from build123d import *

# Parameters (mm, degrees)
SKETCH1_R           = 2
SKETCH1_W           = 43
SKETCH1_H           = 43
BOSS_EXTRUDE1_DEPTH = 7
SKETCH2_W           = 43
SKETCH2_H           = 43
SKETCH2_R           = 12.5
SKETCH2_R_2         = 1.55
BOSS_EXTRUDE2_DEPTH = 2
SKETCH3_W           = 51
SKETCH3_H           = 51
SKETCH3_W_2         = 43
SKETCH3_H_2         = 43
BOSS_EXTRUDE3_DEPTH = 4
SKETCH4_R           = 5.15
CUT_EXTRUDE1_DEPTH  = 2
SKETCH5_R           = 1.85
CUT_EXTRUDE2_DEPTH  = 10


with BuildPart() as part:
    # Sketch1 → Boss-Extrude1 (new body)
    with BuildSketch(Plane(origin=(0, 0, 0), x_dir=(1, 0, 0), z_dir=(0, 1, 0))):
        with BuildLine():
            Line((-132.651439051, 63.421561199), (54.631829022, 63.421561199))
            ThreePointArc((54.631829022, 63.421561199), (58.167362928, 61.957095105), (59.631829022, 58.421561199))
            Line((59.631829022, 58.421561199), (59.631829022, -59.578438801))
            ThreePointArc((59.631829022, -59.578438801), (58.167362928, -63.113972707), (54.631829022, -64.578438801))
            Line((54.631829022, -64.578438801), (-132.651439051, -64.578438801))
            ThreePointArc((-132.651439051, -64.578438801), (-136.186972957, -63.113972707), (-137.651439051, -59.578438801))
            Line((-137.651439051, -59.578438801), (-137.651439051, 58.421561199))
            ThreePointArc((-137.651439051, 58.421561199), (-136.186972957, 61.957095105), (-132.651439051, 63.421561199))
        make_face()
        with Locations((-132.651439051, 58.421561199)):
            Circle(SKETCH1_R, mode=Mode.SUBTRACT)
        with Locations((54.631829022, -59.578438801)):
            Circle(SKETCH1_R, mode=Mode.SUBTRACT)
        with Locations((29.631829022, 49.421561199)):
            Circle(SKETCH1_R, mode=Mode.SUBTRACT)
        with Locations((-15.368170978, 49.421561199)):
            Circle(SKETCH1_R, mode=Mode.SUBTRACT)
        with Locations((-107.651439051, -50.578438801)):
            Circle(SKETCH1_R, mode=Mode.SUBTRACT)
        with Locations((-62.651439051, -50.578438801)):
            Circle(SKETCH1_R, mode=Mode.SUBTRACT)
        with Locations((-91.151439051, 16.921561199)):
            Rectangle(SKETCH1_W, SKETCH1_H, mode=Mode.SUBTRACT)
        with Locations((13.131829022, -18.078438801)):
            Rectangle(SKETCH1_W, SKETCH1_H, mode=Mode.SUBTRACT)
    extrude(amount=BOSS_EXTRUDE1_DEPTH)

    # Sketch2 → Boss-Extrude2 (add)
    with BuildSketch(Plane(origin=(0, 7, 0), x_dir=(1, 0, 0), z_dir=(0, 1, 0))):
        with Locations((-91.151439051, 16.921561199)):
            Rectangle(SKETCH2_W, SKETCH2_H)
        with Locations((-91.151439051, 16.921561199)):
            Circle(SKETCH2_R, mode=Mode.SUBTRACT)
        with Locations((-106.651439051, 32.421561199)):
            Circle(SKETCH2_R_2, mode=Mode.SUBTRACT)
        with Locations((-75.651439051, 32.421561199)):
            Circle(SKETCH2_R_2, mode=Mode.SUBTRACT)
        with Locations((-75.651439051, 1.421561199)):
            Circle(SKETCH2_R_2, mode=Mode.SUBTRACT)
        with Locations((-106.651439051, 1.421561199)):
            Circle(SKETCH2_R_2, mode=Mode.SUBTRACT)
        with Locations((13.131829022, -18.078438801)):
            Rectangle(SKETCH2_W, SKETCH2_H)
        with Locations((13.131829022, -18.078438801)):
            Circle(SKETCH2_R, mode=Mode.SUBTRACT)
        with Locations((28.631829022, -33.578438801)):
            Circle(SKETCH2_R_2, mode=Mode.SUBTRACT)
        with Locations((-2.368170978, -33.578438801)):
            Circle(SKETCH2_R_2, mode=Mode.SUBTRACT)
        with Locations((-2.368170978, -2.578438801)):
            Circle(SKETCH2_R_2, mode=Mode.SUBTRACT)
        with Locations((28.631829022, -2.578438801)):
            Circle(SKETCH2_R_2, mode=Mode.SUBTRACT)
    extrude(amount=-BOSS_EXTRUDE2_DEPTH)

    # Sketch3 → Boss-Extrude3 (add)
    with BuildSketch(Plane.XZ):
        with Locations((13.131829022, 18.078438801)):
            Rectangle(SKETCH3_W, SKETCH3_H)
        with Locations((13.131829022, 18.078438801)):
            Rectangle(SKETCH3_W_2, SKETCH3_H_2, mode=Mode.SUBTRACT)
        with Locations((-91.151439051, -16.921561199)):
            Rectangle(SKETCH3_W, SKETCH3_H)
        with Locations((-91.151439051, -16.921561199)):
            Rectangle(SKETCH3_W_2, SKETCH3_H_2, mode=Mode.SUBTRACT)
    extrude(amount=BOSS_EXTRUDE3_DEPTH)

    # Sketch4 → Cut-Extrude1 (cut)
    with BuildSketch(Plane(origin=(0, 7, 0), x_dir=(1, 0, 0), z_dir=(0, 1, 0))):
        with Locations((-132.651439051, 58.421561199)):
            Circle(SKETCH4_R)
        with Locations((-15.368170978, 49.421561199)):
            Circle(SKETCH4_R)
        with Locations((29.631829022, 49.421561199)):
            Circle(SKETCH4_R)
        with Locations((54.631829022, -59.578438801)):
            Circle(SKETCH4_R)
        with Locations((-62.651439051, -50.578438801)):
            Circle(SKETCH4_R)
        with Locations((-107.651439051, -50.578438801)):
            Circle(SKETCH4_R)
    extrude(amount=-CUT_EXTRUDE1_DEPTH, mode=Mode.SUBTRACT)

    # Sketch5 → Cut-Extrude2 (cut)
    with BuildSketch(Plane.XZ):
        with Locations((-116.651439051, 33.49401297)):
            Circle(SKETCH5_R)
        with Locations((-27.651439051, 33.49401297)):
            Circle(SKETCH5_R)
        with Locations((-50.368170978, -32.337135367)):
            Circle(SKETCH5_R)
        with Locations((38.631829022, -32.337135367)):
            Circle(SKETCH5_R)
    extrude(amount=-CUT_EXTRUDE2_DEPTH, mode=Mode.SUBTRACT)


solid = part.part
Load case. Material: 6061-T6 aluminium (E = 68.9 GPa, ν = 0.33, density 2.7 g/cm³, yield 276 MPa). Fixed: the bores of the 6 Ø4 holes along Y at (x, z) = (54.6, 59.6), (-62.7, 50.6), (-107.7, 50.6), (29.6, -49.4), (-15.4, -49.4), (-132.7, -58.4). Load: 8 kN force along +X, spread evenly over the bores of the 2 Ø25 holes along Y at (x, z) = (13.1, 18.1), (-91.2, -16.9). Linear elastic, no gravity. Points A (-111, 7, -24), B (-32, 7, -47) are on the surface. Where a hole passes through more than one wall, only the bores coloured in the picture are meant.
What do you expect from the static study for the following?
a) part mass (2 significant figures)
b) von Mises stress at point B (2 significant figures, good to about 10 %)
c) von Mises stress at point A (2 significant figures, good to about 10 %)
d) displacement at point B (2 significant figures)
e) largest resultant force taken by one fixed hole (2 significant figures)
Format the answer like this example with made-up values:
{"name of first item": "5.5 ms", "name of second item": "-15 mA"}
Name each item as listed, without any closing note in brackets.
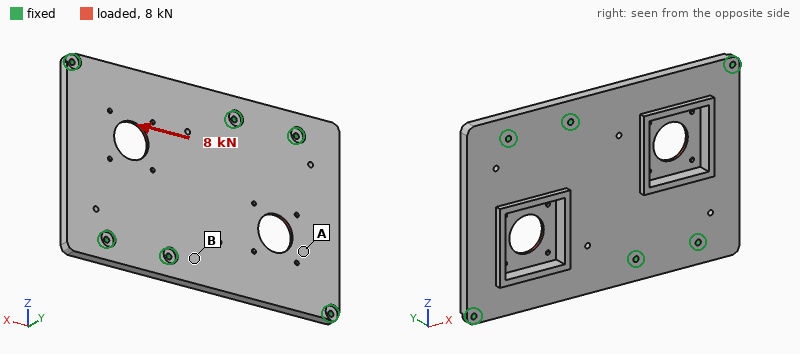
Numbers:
{"part mass": "430 g", "von Mises stress at point B": "7.3 MPa", "von Mises stress at point A": "18 MPa", "displacement at point B": "3.3 µm", "largest resultant force taken by one fixed hole": "1.9 kN"}
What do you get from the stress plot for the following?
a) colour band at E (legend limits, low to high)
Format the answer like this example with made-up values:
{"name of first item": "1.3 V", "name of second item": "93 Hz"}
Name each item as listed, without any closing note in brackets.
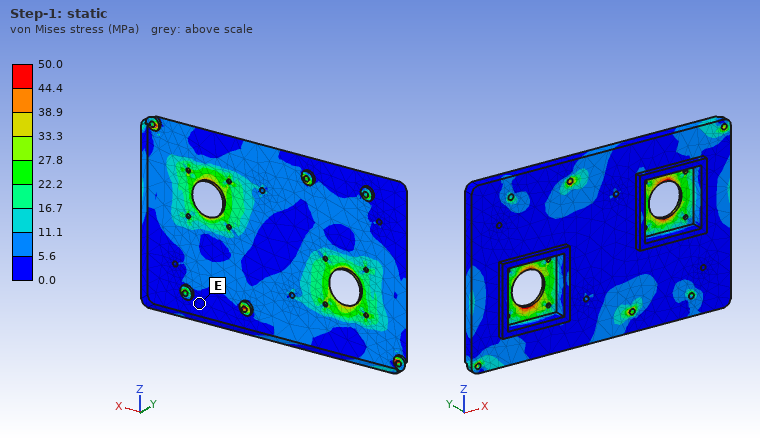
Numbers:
{"colour band at E": "0.0 to 5.6 MPa"}
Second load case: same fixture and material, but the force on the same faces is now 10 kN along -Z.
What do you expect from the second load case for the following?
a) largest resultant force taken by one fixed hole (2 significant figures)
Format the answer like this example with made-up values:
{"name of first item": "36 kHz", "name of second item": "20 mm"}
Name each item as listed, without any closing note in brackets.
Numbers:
{"largest resultant force taken by one fixed hole": "2.0 kN"}
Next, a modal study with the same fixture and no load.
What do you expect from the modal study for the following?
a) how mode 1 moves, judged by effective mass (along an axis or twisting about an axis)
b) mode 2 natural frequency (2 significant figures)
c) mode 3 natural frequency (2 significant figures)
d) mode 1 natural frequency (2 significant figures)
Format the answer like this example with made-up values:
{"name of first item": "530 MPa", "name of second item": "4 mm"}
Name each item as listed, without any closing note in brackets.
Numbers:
{"how mode 1 moves, judged by effective mass": "along Y", "mode 2 natural frequency": "2100 Hz", "mode 3 natural frequency": "2600 Hz", "mode 1 natural frequency": "1900 Hz"}
